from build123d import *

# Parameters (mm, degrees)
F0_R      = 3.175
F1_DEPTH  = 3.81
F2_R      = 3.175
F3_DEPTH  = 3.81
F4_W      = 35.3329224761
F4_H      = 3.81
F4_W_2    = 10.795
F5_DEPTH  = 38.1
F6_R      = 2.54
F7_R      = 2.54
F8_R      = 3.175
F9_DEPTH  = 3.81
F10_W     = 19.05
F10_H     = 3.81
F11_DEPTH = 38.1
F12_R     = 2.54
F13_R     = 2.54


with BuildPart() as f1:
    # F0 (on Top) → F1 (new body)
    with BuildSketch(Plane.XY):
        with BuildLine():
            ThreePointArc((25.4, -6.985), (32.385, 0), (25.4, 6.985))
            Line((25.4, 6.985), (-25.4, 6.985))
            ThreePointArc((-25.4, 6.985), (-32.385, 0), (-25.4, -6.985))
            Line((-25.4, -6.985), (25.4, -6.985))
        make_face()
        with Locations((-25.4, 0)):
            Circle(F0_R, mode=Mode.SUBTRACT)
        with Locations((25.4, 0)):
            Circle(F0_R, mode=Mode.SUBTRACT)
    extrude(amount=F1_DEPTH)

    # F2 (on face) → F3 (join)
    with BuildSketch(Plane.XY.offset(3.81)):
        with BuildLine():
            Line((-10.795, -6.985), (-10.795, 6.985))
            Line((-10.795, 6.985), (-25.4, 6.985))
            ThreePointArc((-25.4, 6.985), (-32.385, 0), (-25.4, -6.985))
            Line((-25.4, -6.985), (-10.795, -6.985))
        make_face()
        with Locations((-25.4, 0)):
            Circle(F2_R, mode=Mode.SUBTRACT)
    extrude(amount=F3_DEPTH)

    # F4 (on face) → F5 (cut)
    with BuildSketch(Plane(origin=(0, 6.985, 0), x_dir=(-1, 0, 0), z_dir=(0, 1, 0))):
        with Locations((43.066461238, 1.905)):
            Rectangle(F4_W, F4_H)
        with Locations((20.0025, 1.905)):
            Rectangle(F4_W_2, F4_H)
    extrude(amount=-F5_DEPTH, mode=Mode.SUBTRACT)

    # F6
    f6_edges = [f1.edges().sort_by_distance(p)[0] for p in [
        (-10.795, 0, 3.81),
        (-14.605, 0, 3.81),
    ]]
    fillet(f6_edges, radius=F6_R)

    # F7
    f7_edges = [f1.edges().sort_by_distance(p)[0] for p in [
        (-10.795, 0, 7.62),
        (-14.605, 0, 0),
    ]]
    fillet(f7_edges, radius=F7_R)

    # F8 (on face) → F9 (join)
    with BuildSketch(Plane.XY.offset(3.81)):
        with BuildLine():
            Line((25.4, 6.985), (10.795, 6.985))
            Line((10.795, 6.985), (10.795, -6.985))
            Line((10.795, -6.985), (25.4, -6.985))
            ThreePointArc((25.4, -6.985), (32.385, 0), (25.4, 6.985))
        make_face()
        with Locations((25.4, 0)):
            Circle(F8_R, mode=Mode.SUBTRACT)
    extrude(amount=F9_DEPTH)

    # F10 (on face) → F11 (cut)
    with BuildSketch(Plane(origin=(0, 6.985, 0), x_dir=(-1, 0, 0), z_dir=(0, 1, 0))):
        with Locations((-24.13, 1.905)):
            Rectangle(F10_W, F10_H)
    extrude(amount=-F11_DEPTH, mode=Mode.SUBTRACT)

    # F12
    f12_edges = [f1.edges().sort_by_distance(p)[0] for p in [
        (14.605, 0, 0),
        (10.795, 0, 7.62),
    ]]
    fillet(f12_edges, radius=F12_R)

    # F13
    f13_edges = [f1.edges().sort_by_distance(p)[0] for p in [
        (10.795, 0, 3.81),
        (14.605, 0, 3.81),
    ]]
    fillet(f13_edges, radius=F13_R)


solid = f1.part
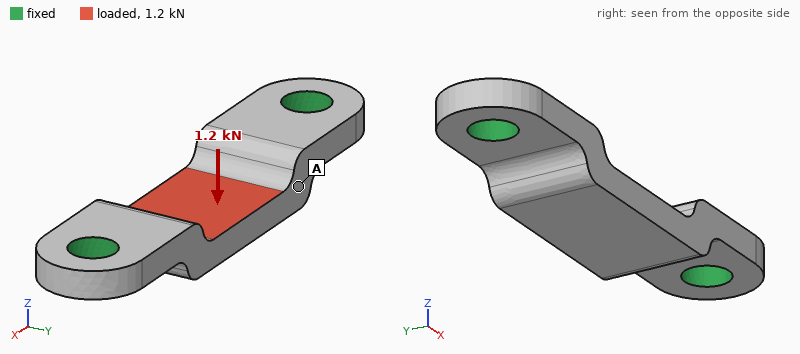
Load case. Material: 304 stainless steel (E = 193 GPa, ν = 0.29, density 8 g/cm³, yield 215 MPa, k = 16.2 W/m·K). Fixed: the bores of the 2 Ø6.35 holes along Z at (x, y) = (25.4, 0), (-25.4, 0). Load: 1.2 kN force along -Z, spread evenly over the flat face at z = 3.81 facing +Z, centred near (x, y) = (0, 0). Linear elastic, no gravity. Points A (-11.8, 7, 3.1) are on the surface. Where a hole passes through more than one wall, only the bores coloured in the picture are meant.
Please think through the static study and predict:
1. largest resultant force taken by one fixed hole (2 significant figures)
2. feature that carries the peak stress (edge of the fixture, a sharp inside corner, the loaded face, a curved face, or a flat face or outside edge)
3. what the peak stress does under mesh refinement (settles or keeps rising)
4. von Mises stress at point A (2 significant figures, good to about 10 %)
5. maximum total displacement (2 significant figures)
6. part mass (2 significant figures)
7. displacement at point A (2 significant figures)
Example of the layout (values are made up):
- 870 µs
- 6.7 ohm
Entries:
- 1.5 kN
- edge of the fixture
- keeps rising
- 30 MPa
- 20 µm
- 28 g
- 10 µm
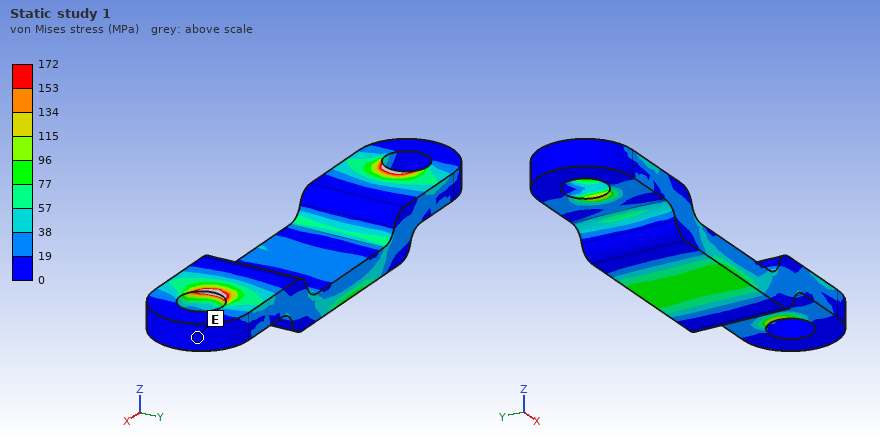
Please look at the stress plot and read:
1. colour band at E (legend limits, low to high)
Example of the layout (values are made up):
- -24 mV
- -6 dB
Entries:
- 0 to 19 MPa
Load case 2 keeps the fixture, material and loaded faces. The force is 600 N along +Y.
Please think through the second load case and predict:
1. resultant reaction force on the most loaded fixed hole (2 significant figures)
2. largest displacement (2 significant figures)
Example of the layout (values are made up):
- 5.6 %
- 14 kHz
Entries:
- 300 N
- 5.2 µm
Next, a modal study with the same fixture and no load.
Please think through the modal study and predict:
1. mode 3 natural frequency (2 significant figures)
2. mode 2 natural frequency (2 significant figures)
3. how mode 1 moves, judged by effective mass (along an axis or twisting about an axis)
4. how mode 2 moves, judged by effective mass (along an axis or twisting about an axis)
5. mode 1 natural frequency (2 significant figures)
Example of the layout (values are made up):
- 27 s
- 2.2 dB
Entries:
- 20 kHz
- 13 kHz
- along Z
- along Y
- 13 kHz
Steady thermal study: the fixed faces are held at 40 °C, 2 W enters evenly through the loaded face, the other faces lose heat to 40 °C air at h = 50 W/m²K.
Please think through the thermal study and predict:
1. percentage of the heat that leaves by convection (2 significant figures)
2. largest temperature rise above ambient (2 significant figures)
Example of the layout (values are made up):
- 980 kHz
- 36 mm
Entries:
- 34 %
- 17 K
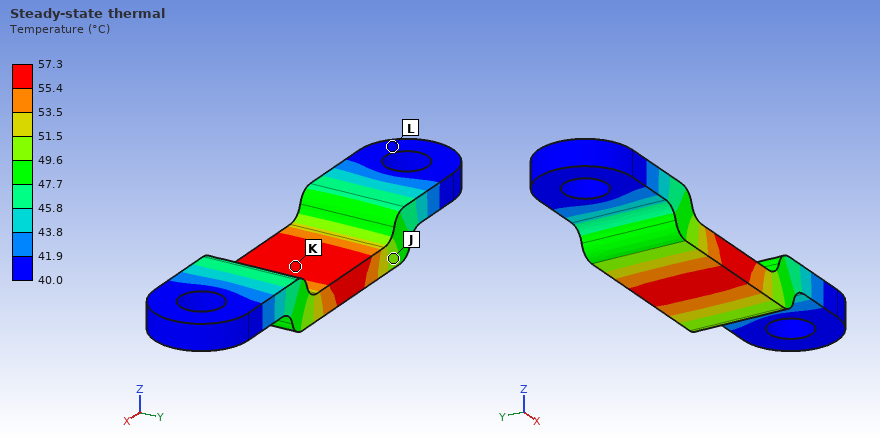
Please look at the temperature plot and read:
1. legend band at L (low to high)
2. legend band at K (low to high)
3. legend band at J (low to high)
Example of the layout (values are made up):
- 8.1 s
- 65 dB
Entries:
- 40.0 to 41.9 °C
- 55.4 to 57.3 °C
- 49.6 to 51.5 °C
